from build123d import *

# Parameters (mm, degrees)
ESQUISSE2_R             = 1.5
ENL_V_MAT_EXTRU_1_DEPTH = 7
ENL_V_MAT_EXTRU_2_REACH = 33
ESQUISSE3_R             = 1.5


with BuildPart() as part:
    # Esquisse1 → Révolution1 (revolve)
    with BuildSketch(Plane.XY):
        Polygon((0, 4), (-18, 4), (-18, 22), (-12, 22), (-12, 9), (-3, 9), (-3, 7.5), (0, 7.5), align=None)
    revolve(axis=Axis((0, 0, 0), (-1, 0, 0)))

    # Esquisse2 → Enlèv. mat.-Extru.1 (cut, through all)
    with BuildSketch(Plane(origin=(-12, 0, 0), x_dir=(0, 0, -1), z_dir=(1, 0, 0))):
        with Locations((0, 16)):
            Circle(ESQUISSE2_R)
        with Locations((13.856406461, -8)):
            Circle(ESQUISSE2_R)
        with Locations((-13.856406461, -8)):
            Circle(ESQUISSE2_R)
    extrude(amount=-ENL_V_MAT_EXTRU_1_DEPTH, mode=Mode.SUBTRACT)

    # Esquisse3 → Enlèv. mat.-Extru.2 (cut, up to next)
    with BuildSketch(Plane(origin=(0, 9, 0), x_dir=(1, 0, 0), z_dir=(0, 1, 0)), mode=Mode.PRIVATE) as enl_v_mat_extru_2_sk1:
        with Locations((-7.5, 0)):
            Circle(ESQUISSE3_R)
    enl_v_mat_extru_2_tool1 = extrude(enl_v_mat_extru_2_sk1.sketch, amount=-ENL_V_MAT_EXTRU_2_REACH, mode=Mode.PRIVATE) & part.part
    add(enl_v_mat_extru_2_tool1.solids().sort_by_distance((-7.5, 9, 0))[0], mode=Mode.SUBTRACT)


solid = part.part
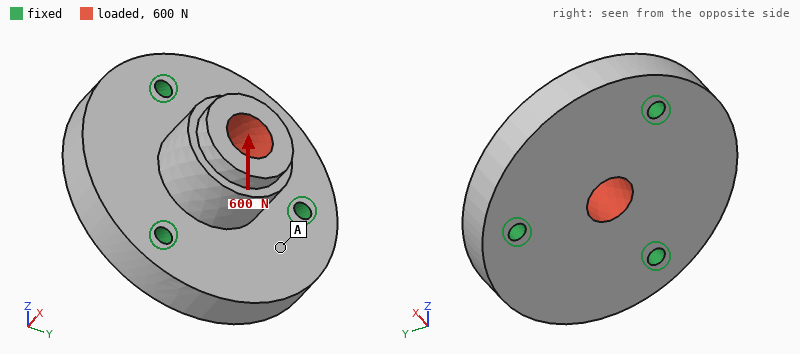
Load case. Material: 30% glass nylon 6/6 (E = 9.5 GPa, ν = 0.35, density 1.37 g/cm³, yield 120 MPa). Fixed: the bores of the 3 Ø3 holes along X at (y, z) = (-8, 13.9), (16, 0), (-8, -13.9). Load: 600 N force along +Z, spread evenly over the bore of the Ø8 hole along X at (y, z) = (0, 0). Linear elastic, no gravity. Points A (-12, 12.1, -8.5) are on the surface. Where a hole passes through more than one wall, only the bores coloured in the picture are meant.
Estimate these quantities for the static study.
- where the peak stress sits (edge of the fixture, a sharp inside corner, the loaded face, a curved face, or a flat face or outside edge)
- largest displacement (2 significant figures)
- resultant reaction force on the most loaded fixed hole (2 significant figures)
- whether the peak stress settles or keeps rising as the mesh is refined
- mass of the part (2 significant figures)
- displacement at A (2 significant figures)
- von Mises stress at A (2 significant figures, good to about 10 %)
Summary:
edge of the fixture
24 µm
250 N
keeps rising
15 g
6.0 µm
1.3 MPa
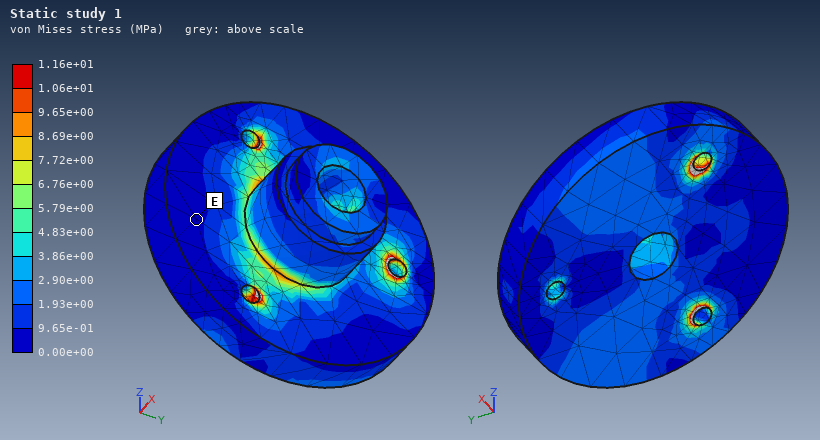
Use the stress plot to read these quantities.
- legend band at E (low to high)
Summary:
0.00e+00 to 9.65e-01 MPa
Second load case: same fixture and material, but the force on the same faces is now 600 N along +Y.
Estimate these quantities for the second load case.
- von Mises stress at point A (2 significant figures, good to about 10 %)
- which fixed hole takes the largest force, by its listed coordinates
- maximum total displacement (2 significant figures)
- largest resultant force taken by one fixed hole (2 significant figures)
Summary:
1.9 MPa
(16, 0)
25 µm
270 N
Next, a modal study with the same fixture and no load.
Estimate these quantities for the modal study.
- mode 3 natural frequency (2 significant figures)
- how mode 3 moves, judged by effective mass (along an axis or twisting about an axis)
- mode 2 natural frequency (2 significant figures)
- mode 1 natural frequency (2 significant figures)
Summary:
11 kHz
along X
9700 Hz
9700 Hz
